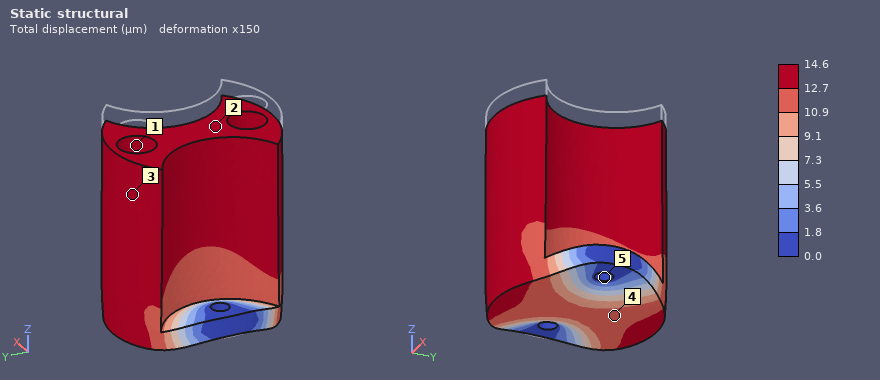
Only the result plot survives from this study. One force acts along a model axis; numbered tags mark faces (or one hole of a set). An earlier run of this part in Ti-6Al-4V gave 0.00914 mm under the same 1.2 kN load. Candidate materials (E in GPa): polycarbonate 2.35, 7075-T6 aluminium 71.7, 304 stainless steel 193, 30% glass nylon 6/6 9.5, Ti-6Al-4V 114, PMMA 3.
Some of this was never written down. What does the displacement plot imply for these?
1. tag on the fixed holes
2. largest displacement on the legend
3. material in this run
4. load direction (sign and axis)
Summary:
5
14.6 µm
7075-T6 aluminium
-Z
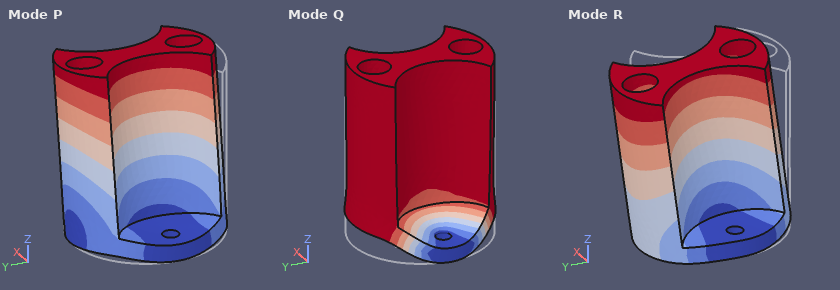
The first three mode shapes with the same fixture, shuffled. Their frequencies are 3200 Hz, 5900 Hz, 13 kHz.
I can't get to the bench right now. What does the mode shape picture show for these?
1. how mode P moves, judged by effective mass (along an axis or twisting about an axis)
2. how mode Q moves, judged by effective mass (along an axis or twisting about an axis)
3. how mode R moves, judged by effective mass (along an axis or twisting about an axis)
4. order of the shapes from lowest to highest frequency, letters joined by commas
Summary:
along X
along Z
along Y
R, P, Q
